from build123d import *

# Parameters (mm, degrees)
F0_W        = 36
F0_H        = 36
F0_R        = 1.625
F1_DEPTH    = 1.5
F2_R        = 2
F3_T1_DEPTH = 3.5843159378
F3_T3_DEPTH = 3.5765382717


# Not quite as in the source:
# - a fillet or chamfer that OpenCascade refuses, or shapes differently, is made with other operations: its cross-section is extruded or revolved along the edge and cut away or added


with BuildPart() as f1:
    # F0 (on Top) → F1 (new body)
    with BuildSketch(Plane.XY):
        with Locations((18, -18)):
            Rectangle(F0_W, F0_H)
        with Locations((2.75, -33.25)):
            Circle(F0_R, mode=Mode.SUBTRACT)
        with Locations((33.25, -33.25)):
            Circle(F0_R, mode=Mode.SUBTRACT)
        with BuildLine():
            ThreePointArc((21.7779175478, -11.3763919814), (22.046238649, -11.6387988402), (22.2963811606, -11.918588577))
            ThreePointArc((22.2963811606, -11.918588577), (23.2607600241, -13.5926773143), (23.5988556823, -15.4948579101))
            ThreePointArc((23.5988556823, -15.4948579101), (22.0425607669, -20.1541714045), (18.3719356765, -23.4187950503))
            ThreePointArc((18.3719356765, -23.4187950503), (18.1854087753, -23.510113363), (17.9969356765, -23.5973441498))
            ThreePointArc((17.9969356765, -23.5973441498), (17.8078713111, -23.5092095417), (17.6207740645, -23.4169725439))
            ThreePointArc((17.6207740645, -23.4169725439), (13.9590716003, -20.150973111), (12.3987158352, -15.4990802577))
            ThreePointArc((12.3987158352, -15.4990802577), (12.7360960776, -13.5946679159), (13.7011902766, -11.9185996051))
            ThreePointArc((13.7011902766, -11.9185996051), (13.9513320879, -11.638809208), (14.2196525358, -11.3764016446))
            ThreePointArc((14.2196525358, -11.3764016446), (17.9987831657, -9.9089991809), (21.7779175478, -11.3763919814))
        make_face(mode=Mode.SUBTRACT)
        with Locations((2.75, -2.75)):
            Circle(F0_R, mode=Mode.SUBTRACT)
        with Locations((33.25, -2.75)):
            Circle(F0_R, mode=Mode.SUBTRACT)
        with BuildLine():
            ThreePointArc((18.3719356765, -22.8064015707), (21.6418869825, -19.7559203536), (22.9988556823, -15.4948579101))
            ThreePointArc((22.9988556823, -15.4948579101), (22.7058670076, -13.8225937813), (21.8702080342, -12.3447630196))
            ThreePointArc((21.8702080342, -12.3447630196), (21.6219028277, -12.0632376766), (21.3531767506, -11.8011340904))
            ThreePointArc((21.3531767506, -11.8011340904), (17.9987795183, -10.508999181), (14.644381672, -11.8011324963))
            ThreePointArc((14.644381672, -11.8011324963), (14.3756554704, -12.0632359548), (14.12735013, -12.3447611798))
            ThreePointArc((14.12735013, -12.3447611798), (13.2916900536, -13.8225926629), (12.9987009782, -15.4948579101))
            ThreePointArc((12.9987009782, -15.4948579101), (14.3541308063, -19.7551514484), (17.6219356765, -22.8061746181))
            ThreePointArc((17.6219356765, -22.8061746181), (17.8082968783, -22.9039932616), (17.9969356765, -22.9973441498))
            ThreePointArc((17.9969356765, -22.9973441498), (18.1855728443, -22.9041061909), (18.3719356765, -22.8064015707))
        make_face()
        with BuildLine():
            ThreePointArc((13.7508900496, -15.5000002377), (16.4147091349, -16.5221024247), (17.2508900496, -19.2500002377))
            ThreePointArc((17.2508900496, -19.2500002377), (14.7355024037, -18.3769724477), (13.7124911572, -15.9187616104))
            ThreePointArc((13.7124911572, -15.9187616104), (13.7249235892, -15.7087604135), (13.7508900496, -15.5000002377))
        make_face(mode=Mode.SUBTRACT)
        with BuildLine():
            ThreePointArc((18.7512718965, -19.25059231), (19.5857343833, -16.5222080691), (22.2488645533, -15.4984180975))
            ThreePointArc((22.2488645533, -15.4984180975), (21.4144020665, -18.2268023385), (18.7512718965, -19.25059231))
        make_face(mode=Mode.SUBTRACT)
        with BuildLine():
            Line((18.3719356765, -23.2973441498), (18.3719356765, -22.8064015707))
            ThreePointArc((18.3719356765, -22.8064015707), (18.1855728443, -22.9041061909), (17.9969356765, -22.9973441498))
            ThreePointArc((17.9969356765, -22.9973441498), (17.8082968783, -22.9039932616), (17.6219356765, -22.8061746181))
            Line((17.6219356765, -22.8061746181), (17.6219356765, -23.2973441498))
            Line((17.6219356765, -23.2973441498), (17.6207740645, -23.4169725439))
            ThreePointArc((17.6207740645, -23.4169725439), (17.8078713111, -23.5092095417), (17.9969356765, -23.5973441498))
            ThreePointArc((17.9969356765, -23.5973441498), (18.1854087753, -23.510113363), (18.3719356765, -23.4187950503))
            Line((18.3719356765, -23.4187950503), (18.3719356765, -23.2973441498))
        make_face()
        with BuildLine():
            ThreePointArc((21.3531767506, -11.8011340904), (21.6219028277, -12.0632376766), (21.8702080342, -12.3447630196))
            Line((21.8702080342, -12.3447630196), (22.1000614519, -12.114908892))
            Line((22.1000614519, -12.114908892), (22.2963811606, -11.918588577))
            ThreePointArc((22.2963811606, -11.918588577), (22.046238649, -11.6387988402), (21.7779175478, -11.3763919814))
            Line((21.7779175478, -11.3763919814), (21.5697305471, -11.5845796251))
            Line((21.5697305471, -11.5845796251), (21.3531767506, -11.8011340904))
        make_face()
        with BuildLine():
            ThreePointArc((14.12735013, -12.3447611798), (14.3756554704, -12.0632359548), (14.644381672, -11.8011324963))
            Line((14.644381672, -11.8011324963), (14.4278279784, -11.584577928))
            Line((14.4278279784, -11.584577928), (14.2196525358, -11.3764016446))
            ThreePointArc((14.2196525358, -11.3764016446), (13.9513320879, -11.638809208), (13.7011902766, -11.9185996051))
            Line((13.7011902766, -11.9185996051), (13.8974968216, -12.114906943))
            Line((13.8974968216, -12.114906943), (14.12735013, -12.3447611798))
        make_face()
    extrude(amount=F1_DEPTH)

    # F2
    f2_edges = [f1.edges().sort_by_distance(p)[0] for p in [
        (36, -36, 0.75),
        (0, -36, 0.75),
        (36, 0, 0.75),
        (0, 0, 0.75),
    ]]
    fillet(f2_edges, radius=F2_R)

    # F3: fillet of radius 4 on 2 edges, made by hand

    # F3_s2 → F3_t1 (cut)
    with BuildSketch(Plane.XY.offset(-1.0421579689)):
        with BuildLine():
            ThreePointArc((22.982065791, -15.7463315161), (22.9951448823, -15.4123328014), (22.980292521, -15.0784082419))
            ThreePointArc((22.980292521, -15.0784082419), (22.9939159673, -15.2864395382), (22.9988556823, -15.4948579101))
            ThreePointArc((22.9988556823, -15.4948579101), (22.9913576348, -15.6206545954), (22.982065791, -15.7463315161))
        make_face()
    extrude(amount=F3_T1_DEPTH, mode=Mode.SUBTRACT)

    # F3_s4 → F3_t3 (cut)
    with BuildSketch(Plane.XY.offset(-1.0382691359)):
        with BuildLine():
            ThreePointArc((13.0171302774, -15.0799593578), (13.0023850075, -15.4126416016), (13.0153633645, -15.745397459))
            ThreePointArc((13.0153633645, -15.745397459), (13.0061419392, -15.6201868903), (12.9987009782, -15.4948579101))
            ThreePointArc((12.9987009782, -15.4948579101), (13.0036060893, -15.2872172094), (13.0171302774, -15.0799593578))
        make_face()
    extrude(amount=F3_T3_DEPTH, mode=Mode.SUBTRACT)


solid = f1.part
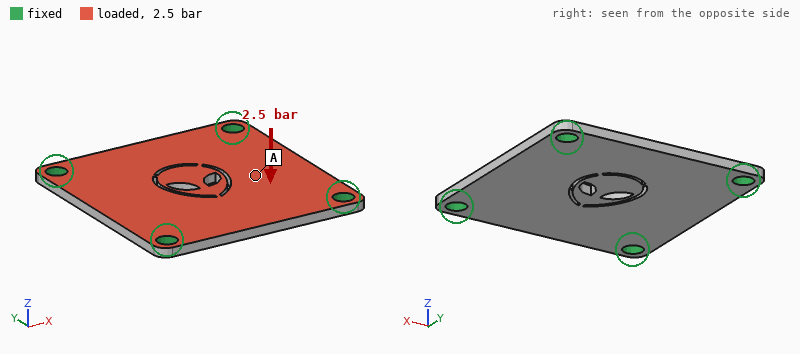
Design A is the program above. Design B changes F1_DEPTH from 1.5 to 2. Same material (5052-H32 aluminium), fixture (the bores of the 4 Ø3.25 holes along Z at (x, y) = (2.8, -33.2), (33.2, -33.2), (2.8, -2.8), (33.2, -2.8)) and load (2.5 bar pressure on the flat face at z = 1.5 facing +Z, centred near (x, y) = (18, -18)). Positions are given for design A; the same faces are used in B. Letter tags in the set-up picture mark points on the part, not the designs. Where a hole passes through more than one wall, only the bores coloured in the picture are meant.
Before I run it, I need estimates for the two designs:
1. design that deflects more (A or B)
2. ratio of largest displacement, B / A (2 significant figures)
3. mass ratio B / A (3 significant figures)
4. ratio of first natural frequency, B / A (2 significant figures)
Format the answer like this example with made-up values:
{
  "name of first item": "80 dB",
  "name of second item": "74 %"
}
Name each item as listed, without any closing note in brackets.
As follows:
{
  "design that deflects more": "A",
  "ratio of largest displacement, B / A": "0.45",
  "mass ratio B / A": "1.33",
  "ratio of first natural frequency, B / A": "1.3"
}
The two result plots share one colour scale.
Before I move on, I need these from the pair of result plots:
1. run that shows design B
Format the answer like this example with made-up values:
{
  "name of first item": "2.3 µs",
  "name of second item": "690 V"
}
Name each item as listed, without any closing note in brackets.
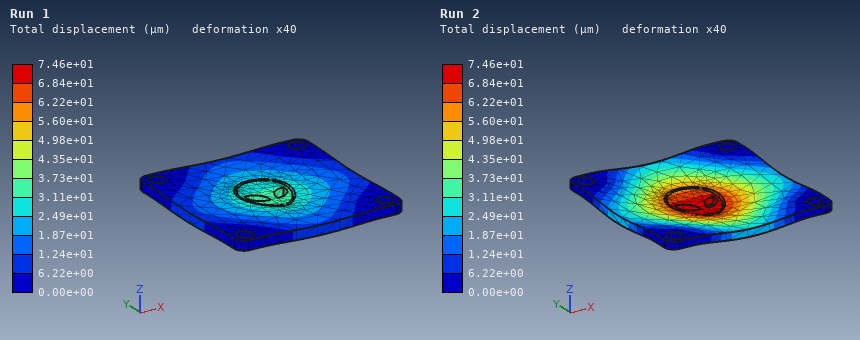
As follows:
{
  "run that shows design B": "Run 1"
}
